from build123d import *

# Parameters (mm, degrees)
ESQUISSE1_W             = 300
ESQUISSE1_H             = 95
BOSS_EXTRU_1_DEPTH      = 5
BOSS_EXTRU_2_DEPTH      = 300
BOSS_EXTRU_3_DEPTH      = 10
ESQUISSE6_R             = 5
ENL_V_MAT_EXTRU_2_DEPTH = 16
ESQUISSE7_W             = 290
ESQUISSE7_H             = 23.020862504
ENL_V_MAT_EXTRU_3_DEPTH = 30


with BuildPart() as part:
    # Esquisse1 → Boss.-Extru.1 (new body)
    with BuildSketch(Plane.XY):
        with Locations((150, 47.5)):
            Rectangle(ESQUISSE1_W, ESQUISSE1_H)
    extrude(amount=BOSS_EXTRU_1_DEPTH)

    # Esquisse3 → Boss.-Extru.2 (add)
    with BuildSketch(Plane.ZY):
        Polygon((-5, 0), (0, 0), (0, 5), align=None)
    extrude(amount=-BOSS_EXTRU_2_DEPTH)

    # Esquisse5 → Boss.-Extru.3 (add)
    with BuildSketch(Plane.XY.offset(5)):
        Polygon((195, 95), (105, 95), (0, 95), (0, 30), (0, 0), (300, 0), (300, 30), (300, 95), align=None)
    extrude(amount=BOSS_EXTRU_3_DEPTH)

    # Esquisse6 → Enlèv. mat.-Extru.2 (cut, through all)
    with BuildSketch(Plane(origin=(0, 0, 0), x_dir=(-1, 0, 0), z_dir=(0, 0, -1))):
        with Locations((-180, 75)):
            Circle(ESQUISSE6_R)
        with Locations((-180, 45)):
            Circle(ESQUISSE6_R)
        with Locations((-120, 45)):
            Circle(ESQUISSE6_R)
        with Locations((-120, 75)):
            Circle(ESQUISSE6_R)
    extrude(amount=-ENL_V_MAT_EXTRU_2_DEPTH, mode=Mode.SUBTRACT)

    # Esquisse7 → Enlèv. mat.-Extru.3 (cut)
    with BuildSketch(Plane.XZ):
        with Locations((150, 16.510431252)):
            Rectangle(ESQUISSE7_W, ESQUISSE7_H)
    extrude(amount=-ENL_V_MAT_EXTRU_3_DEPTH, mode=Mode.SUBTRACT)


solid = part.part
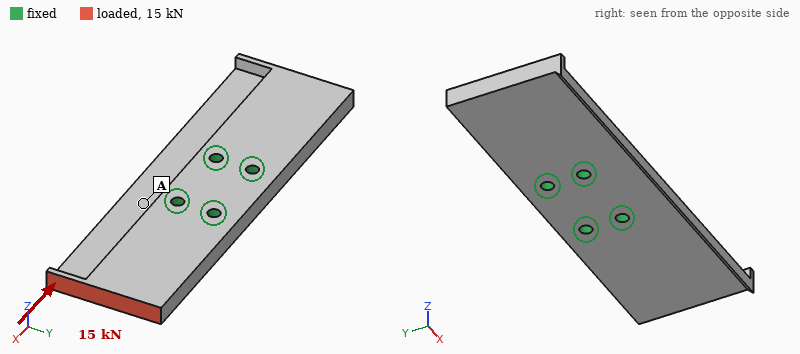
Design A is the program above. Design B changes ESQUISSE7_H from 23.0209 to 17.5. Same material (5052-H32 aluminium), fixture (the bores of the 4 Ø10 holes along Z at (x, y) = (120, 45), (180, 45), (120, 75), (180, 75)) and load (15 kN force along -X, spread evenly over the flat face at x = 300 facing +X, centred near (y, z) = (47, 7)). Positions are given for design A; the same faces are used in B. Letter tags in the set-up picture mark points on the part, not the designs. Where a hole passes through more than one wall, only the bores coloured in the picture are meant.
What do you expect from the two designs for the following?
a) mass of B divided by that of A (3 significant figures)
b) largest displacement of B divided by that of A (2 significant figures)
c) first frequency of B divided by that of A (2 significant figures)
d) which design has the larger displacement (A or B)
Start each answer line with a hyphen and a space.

- 1.07
- 0.60
- 0.98
- A
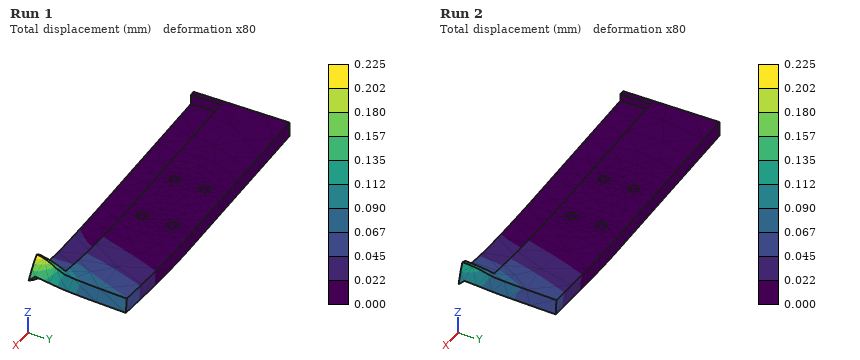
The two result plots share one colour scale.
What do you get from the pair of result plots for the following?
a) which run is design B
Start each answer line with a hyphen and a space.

- Run 2
